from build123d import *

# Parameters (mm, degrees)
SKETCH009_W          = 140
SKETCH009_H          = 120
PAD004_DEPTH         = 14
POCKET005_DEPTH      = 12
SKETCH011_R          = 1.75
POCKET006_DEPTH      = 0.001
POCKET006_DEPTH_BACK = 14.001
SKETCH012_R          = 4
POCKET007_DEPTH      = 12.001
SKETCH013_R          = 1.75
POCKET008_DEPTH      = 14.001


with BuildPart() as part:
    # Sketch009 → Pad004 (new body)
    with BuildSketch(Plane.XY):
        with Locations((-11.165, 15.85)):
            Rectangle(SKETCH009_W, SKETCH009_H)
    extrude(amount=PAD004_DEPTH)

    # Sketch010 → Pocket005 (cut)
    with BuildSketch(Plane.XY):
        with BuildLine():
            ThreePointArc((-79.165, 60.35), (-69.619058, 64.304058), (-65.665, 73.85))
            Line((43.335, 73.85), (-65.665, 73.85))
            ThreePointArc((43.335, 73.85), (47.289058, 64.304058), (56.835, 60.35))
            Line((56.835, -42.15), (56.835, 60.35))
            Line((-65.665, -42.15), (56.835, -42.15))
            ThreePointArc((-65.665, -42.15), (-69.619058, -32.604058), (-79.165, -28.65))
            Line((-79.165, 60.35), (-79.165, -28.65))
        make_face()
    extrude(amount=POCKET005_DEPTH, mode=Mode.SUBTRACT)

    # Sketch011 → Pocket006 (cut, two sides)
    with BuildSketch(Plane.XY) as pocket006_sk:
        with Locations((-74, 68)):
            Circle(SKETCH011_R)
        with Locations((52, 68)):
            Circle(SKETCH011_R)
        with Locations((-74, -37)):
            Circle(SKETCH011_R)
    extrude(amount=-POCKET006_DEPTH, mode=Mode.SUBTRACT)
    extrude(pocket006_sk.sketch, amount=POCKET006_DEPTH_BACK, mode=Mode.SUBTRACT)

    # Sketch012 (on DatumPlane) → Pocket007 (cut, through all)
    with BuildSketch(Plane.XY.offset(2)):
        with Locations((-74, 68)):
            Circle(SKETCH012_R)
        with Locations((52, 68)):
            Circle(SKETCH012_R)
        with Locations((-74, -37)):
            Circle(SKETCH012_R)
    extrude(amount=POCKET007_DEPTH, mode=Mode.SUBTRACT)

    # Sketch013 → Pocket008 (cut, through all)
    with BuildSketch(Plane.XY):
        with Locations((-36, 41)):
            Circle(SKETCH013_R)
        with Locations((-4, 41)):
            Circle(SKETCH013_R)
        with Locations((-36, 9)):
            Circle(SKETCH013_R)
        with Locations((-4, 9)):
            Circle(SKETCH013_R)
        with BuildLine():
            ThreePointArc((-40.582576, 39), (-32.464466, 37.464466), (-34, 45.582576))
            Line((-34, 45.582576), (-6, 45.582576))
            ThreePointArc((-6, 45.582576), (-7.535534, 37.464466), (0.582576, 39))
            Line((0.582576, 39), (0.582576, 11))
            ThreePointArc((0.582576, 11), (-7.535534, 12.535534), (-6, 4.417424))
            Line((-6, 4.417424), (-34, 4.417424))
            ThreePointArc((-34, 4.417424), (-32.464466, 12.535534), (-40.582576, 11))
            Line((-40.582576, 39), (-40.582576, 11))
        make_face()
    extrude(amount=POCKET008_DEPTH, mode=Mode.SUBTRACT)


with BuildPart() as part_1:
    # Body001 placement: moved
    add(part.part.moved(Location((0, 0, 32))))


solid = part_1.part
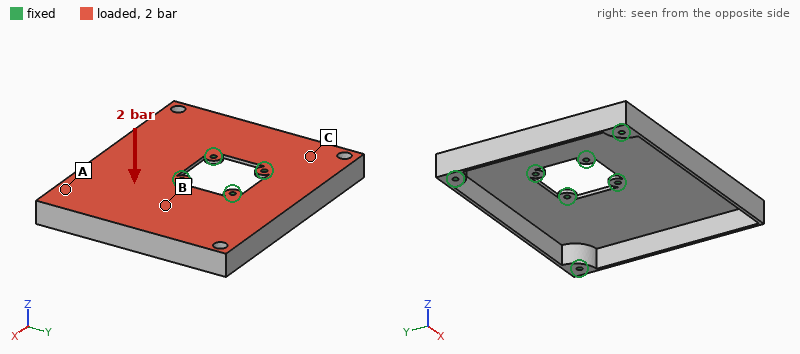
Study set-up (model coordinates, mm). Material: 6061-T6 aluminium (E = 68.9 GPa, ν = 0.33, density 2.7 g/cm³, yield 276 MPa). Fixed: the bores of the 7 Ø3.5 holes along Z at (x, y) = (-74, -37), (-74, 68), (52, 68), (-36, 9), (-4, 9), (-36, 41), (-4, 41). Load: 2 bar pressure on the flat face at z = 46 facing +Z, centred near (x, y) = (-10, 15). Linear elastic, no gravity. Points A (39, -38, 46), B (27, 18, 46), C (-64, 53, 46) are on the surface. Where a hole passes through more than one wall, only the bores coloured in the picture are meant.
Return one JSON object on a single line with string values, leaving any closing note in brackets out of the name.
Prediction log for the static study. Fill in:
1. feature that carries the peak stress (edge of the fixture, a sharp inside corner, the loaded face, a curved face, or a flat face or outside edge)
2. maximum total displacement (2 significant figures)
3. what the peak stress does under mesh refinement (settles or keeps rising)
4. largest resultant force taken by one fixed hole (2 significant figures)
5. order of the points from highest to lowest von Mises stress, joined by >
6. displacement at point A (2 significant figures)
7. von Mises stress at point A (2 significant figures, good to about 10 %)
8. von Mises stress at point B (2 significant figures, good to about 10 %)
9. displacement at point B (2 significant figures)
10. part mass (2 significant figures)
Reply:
{"feature that carries the peak stress": "edge of the fixture", "maximum total displacement": "1.2 mm", "what the peak stress does under mesh refinement": "keeps rising", "largest resultant force taken by one fixed hole": "2.3 kN", "order of the points from highest to lowest von Mises stress, joined by >": "B > A > C", "displacement at point A": "1.00 mm", "von Mises stress at point A": "41 MPa", "von Mises stress at point B": "68 MPa", "displacement at point B": "0.48 mm", "part mass": "130 g"}
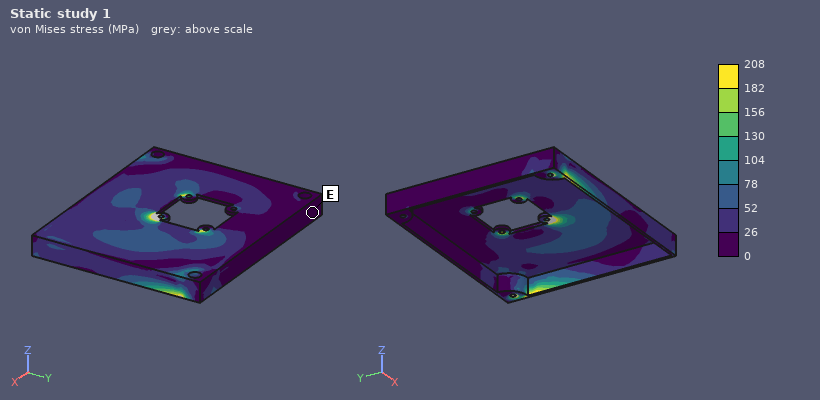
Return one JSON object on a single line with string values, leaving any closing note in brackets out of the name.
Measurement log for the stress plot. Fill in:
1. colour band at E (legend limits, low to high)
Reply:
{"colour band at E": "0 to 26 MPa"}
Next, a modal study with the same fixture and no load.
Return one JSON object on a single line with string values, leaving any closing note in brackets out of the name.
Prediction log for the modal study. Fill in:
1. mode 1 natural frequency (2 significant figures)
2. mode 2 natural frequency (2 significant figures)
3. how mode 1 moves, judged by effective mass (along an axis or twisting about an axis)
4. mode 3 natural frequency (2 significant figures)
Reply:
{"mode 1 natural frequency": "910 Hz", "mode 2 natural frequency": "2200 Hz", "how mode 1 moves, judged by effective mass": "along Z", "mode 3 natural frequency": "2400 Hz"}
